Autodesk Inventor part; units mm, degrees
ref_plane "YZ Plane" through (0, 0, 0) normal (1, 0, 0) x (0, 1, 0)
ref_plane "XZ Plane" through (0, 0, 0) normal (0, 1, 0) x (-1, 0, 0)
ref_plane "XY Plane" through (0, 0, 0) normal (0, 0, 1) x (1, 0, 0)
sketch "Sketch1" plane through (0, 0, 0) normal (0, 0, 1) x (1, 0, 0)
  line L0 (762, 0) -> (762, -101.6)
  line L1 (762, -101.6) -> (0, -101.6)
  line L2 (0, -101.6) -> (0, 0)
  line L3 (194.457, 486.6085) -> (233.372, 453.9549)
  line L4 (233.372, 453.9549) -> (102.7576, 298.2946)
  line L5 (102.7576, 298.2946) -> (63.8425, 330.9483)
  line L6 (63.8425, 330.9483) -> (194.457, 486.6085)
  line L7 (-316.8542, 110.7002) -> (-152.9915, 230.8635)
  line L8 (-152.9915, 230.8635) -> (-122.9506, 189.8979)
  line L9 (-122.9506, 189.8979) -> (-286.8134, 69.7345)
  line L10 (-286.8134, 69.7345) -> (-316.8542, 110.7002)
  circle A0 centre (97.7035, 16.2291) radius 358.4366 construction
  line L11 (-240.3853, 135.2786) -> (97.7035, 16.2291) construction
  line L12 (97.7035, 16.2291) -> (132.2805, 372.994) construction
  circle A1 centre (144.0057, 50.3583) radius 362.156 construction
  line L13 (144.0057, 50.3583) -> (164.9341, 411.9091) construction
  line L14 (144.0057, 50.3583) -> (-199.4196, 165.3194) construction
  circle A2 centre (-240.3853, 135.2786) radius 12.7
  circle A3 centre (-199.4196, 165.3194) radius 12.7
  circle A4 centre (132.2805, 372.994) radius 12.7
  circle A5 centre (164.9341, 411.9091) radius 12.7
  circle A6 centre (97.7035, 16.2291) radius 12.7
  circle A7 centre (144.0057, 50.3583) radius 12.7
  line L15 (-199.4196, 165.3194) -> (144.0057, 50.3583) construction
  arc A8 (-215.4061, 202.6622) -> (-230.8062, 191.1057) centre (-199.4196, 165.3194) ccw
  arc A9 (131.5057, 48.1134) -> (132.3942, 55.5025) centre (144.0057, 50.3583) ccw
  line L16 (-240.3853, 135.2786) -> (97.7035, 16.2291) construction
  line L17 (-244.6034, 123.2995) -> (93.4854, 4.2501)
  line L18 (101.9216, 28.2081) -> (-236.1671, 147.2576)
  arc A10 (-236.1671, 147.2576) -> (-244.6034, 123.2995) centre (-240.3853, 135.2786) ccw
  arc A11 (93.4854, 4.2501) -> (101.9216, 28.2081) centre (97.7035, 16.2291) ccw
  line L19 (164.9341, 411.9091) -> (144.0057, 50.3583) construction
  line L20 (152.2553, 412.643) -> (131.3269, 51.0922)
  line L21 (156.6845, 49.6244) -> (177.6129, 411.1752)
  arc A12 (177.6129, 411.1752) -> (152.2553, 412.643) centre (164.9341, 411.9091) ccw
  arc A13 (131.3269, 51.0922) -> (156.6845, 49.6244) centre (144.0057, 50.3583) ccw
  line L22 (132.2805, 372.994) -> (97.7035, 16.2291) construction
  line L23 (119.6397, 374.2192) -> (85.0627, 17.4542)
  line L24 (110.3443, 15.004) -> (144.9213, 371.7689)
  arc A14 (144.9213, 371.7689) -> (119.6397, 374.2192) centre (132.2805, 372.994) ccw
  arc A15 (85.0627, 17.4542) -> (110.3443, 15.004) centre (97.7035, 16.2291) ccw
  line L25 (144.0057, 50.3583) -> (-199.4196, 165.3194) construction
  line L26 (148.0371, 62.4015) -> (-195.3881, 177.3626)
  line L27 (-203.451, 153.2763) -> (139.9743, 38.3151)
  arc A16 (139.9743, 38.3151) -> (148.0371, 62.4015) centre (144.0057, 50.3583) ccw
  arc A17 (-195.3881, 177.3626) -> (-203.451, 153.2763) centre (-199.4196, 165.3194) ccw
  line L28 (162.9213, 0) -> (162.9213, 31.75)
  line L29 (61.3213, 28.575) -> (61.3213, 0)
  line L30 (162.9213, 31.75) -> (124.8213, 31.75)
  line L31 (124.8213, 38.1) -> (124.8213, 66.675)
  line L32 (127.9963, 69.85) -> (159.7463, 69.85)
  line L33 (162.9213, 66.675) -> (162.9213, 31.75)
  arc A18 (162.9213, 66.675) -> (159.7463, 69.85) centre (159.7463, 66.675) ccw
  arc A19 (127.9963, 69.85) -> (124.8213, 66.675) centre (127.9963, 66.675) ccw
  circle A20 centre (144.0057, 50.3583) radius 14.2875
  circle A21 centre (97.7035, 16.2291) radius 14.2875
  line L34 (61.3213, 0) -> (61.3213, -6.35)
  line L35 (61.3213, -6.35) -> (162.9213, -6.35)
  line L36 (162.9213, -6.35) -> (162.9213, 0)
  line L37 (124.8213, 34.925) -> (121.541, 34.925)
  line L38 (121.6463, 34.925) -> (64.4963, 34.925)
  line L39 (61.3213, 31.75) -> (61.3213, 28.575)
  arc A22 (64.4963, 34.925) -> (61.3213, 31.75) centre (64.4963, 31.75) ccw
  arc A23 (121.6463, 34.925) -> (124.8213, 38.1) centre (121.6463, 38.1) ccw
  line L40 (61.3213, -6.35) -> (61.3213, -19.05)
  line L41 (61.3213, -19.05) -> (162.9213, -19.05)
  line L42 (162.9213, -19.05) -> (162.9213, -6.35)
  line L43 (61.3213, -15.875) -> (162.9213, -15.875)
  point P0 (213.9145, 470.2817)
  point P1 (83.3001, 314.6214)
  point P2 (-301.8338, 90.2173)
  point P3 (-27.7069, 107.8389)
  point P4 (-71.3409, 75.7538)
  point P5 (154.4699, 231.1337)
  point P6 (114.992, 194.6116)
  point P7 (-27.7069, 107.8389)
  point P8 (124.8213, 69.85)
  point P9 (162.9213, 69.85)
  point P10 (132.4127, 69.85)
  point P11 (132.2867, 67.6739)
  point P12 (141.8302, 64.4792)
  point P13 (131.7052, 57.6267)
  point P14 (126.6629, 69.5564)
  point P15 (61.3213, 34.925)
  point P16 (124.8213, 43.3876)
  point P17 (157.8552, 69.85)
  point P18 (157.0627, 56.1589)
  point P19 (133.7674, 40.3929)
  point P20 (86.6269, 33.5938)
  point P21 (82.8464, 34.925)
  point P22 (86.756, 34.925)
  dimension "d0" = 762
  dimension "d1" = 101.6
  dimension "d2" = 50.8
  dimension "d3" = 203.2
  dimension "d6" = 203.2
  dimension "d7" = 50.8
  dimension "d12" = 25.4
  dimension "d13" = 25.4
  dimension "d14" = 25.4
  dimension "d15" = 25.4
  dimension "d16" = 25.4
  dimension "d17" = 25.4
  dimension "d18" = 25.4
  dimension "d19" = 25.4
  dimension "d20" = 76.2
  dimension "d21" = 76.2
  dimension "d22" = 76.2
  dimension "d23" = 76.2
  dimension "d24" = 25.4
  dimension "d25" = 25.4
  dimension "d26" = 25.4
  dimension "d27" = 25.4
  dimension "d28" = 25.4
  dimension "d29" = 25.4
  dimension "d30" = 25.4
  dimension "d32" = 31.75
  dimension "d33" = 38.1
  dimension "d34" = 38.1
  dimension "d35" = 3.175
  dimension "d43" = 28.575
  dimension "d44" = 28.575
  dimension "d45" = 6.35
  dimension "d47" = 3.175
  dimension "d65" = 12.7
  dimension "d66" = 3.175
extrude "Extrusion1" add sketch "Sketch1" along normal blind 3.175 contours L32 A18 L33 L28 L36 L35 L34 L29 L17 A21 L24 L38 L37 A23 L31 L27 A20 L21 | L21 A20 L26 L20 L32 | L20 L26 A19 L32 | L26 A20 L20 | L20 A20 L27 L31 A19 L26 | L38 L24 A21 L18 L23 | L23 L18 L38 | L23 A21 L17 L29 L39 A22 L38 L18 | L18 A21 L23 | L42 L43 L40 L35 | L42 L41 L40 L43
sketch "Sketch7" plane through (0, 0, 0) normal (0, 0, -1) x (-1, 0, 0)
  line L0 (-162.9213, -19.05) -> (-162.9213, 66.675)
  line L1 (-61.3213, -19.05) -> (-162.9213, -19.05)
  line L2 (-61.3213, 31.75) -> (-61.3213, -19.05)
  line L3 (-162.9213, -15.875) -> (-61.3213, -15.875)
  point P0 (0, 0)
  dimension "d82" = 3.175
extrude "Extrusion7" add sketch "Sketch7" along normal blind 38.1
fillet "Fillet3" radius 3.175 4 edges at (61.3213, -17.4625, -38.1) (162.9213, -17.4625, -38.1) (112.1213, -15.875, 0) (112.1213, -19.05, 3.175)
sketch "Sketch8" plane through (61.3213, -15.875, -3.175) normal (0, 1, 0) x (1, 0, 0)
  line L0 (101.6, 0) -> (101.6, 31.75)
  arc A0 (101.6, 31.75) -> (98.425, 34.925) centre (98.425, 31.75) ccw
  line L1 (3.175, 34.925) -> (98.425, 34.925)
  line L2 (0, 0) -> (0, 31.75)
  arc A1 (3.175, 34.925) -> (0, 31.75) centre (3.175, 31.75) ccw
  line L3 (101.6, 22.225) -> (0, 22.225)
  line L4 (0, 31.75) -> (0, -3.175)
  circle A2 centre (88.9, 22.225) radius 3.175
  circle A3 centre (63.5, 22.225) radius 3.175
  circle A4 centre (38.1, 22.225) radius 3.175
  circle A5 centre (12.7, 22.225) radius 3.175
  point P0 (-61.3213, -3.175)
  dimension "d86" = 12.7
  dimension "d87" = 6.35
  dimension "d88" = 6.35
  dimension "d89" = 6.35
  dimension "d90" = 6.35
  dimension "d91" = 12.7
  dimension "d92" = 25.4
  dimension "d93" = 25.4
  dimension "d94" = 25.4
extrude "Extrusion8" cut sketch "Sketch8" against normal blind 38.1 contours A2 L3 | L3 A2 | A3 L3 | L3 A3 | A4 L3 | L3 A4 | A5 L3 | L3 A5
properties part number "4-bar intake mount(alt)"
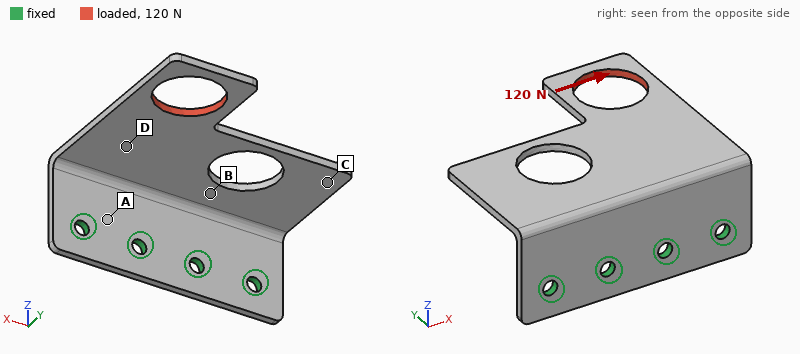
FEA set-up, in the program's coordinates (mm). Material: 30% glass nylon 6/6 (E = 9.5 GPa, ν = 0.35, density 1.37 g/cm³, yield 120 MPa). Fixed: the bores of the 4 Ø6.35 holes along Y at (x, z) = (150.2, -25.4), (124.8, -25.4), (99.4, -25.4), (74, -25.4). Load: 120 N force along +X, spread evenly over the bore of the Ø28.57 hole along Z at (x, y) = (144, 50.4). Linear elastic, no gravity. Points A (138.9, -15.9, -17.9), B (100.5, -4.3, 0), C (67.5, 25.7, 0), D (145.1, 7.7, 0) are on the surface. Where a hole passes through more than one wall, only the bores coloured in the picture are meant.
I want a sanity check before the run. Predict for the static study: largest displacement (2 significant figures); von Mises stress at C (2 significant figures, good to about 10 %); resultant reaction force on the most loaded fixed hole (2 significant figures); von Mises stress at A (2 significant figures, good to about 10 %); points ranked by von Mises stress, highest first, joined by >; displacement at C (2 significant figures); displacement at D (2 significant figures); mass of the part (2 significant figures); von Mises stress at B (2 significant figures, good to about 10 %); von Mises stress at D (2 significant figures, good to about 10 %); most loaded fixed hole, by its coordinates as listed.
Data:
1.4 mm
2.9 MPa
110 N
13 MPa
A > B > D > C
0.78 mm
0.49 mm
40 g
10 MPa
4.7 MPa
(74, -25.4)
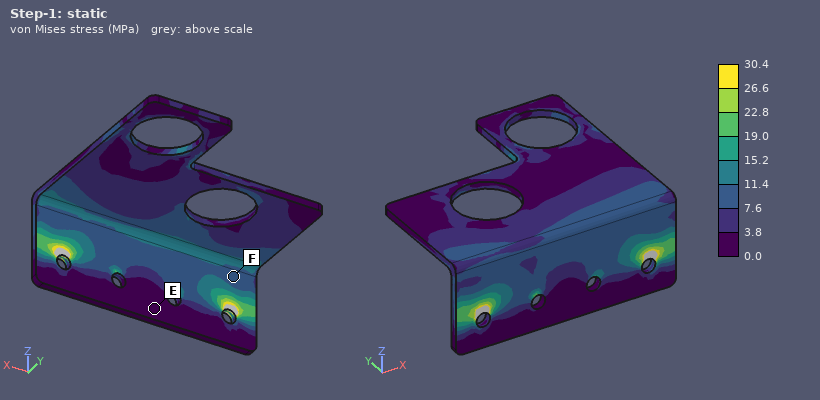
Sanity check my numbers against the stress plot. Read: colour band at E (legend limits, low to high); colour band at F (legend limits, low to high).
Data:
0.0 to 3.8 MPa
7.6 to 11.4 MPa
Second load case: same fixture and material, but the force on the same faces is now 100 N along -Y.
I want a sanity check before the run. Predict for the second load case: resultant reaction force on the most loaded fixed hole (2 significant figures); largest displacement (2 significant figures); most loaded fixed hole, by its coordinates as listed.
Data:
62 N
1.5 mm
(150.2, -25.4)
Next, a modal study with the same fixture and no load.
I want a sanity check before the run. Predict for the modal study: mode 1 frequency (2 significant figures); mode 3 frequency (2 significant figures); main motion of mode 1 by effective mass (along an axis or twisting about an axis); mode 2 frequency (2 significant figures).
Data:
210 Hz
630 Hz
along Z
460 Hz
